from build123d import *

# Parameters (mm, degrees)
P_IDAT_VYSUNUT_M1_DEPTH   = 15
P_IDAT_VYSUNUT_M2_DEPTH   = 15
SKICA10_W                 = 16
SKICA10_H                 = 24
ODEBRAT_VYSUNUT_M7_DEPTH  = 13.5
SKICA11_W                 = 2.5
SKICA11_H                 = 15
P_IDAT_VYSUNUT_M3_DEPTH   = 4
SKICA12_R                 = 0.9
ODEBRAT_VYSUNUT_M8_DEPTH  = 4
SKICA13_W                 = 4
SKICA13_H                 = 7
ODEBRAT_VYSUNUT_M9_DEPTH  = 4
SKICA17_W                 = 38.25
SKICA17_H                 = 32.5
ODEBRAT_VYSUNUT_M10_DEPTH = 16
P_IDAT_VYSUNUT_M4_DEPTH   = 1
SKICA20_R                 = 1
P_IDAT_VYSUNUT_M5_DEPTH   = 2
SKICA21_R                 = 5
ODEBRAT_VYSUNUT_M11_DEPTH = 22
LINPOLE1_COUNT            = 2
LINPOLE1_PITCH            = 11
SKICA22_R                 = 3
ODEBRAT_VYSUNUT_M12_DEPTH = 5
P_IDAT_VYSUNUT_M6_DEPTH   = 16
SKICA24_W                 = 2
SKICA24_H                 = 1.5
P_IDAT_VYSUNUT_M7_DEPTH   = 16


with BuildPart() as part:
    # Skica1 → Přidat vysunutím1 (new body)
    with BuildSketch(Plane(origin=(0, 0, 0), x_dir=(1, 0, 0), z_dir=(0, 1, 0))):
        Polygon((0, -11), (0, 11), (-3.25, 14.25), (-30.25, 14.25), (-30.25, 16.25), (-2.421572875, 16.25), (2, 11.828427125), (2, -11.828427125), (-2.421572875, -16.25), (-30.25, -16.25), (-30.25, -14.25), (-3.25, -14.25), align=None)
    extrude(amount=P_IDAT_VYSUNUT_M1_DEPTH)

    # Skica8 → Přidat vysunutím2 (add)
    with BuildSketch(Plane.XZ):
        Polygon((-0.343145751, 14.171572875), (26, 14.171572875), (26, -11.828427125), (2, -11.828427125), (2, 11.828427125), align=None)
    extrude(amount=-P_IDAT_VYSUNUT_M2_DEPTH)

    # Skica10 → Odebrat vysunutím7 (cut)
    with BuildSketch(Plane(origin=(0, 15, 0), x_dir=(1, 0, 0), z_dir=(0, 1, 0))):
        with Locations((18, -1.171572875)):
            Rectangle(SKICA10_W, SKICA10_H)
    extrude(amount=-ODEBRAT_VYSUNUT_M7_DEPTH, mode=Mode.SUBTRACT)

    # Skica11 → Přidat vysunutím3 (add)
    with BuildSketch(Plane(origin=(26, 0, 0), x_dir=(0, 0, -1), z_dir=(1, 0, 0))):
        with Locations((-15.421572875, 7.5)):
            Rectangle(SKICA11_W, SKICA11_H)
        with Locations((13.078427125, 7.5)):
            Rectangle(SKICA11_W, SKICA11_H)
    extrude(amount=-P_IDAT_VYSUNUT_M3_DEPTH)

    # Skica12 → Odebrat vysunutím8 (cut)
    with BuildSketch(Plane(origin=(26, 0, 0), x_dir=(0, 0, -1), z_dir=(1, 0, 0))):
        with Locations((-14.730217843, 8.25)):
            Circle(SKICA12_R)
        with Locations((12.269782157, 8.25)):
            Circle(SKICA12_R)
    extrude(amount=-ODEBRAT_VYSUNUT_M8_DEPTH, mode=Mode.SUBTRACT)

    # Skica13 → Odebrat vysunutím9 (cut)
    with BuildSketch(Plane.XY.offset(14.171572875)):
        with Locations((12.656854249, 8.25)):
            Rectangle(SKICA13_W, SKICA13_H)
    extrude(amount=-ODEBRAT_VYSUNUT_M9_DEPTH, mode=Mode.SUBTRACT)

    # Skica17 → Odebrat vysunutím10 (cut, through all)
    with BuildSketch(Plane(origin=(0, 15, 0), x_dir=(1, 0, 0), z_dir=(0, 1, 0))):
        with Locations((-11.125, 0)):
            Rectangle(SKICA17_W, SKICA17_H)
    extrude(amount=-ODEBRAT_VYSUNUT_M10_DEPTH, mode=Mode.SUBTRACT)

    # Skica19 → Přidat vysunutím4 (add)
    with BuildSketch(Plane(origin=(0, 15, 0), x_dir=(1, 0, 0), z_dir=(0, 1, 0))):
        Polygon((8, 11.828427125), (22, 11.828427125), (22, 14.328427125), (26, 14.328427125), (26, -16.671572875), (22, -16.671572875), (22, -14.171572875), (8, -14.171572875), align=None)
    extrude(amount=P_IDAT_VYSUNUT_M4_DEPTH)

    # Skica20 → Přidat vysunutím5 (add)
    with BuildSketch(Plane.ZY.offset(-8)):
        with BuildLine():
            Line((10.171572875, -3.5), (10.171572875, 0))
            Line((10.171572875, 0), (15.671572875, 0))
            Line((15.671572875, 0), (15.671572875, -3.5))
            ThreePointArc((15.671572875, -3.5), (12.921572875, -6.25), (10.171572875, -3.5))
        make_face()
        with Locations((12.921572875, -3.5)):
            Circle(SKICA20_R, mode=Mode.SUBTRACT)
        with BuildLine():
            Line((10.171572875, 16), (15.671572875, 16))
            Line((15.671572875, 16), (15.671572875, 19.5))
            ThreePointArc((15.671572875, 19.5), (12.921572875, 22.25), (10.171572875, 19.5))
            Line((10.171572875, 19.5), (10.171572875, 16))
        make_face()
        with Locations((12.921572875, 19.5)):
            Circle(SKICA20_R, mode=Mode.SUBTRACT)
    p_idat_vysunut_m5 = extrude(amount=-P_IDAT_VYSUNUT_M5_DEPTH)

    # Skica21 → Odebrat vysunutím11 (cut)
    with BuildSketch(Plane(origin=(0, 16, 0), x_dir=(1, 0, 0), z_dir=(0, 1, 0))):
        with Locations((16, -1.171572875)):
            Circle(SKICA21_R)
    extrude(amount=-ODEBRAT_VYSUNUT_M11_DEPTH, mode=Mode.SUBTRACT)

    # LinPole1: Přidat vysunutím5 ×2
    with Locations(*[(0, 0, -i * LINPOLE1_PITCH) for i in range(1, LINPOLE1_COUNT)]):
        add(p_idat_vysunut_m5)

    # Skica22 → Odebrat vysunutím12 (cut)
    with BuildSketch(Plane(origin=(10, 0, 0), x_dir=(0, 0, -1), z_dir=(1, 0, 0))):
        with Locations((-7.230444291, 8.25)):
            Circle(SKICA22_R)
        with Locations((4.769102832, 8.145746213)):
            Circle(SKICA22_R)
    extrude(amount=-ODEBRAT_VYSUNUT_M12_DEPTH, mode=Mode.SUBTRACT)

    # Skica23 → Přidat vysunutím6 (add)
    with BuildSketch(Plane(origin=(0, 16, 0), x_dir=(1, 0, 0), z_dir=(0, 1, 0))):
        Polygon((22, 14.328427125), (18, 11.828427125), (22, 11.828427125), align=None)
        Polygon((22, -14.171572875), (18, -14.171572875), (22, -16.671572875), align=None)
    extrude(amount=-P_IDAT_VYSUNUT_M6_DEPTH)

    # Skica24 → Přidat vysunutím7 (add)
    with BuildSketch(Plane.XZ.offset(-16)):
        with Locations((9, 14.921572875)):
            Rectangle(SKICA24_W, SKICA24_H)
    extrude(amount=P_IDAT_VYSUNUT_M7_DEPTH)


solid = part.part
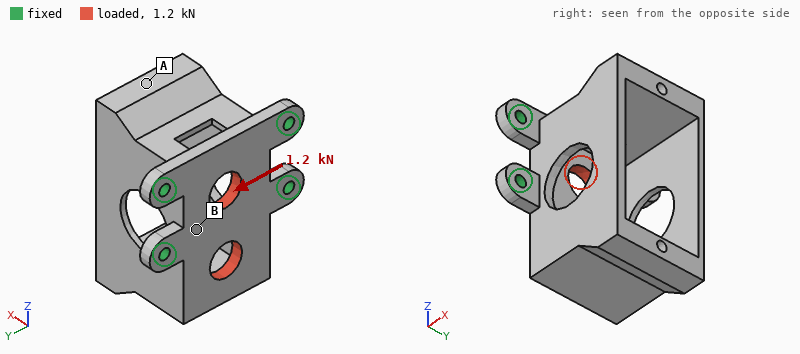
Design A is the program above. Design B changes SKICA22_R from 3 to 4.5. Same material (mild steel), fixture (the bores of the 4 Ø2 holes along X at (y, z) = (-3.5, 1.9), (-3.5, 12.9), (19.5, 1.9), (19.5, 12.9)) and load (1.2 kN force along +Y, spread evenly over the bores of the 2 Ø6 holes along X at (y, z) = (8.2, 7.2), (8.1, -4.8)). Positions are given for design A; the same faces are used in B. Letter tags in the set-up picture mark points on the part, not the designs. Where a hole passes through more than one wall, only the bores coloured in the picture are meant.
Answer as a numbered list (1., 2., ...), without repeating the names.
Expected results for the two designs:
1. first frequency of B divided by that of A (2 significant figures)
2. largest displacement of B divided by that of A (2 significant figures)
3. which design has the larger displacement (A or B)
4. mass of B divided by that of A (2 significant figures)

1. 1.0
2. 1.8
3. B
4. 0.95
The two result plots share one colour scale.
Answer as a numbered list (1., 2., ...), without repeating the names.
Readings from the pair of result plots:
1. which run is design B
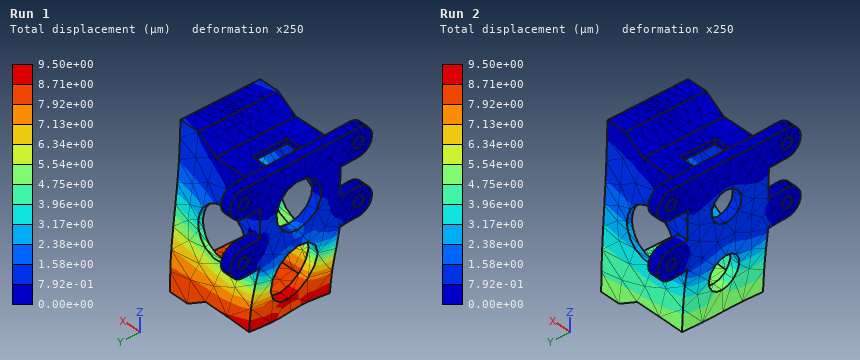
1. Run 1
